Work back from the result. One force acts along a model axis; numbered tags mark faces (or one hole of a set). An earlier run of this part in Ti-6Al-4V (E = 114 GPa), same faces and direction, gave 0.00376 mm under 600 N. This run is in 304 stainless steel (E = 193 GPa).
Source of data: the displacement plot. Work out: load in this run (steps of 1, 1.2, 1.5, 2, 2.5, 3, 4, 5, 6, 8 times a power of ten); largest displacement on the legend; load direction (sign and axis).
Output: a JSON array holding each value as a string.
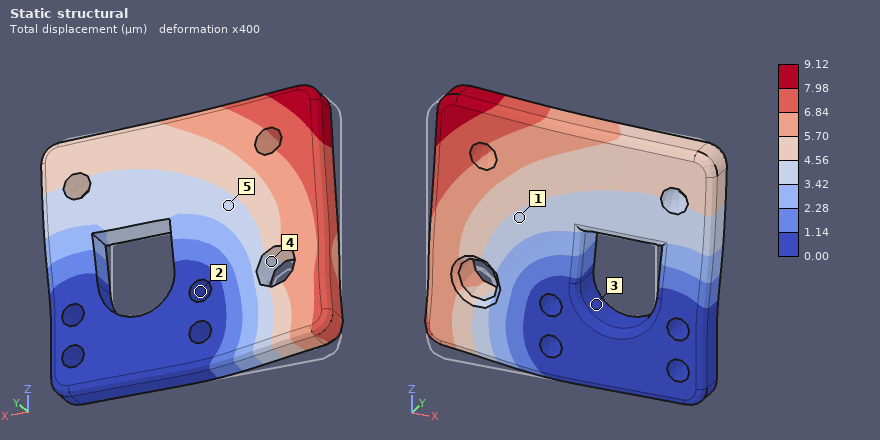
["2.5 kN", "9.12 µm", "+Z"]
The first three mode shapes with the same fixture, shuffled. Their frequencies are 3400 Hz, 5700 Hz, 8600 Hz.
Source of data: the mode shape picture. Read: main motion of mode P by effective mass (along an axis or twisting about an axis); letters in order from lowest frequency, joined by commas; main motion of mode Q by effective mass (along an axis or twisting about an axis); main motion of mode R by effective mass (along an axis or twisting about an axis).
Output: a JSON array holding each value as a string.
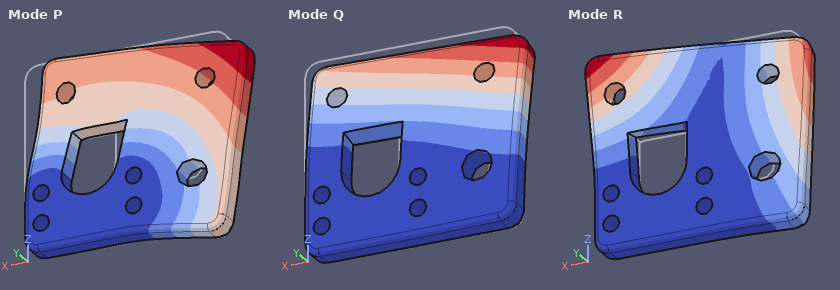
["along X", "Q, R, P", "along Y", "twisting about Z"]
